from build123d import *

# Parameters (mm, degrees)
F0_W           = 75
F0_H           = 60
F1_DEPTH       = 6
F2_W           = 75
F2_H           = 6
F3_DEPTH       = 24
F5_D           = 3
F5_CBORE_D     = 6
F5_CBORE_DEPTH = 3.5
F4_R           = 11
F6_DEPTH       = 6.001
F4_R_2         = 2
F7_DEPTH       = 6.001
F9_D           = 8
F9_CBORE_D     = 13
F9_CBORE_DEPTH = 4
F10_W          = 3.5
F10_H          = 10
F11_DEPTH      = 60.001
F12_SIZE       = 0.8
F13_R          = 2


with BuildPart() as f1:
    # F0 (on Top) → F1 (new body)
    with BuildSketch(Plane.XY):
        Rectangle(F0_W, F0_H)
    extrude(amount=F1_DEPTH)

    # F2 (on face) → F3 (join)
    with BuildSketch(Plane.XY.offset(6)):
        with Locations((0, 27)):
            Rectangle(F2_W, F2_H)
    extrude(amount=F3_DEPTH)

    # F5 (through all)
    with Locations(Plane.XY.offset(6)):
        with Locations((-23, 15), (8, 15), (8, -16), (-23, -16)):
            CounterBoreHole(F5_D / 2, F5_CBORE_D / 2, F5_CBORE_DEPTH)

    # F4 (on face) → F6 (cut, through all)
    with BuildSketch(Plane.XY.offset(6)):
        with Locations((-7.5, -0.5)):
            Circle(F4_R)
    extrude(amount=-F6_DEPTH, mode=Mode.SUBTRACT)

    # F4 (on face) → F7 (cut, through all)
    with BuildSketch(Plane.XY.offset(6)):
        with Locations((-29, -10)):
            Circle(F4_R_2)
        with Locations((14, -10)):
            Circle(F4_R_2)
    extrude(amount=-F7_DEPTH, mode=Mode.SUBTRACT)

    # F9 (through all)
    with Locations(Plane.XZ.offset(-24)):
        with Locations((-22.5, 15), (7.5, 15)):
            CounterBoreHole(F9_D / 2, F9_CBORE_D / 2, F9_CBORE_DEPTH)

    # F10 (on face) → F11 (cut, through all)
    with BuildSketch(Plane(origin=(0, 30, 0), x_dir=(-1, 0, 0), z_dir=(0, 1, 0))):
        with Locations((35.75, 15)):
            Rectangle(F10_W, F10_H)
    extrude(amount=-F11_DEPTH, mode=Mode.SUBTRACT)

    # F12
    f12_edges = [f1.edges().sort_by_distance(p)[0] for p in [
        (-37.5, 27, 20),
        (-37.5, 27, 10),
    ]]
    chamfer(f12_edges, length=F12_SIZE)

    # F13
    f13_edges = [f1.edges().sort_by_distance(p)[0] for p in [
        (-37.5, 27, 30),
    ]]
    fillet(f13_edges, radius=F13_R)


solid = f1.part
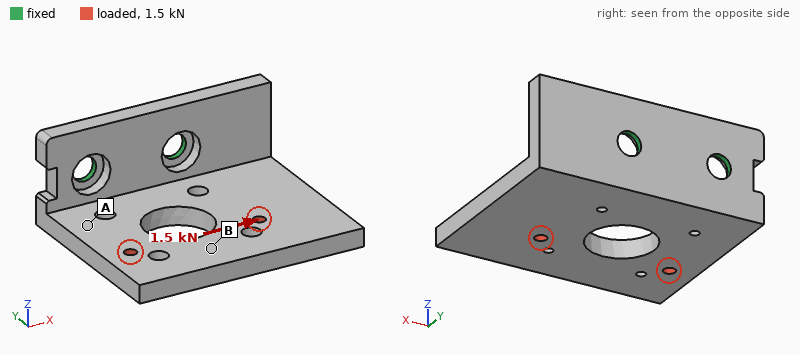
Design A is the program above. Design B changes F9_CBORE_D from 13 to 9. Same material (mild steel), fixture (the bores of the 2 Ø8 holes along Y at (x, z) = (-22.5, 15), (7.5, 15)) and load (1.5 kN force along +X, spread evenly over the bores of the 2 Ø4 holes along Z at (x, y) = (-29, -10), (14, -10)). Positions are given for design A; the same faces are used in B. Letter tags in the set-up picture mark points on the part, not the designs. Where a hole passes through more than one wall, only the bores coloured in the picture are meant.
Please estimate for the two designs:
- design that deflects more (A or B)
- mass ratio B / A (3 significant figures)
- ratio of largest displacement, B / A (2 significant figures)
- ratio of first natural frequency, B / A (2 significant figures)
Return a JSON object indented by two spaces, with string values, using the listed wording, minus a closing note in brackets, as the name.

{
  "design that deflects more": "A",
  "mass ratio B / A": "1.02",
  "ratio of largest displacement, B / A": "0.82",
  "ratio of first natural frequency, B / A": "1.1"
}
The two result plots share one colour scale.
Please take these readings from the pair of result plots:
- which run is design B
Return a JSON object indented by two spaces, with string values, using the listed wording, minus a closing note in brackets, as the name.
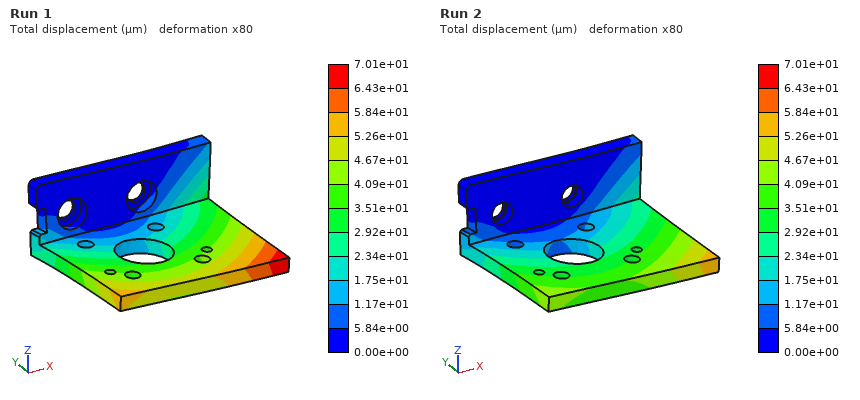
{
  "which run is design B": "Run 2"
}
